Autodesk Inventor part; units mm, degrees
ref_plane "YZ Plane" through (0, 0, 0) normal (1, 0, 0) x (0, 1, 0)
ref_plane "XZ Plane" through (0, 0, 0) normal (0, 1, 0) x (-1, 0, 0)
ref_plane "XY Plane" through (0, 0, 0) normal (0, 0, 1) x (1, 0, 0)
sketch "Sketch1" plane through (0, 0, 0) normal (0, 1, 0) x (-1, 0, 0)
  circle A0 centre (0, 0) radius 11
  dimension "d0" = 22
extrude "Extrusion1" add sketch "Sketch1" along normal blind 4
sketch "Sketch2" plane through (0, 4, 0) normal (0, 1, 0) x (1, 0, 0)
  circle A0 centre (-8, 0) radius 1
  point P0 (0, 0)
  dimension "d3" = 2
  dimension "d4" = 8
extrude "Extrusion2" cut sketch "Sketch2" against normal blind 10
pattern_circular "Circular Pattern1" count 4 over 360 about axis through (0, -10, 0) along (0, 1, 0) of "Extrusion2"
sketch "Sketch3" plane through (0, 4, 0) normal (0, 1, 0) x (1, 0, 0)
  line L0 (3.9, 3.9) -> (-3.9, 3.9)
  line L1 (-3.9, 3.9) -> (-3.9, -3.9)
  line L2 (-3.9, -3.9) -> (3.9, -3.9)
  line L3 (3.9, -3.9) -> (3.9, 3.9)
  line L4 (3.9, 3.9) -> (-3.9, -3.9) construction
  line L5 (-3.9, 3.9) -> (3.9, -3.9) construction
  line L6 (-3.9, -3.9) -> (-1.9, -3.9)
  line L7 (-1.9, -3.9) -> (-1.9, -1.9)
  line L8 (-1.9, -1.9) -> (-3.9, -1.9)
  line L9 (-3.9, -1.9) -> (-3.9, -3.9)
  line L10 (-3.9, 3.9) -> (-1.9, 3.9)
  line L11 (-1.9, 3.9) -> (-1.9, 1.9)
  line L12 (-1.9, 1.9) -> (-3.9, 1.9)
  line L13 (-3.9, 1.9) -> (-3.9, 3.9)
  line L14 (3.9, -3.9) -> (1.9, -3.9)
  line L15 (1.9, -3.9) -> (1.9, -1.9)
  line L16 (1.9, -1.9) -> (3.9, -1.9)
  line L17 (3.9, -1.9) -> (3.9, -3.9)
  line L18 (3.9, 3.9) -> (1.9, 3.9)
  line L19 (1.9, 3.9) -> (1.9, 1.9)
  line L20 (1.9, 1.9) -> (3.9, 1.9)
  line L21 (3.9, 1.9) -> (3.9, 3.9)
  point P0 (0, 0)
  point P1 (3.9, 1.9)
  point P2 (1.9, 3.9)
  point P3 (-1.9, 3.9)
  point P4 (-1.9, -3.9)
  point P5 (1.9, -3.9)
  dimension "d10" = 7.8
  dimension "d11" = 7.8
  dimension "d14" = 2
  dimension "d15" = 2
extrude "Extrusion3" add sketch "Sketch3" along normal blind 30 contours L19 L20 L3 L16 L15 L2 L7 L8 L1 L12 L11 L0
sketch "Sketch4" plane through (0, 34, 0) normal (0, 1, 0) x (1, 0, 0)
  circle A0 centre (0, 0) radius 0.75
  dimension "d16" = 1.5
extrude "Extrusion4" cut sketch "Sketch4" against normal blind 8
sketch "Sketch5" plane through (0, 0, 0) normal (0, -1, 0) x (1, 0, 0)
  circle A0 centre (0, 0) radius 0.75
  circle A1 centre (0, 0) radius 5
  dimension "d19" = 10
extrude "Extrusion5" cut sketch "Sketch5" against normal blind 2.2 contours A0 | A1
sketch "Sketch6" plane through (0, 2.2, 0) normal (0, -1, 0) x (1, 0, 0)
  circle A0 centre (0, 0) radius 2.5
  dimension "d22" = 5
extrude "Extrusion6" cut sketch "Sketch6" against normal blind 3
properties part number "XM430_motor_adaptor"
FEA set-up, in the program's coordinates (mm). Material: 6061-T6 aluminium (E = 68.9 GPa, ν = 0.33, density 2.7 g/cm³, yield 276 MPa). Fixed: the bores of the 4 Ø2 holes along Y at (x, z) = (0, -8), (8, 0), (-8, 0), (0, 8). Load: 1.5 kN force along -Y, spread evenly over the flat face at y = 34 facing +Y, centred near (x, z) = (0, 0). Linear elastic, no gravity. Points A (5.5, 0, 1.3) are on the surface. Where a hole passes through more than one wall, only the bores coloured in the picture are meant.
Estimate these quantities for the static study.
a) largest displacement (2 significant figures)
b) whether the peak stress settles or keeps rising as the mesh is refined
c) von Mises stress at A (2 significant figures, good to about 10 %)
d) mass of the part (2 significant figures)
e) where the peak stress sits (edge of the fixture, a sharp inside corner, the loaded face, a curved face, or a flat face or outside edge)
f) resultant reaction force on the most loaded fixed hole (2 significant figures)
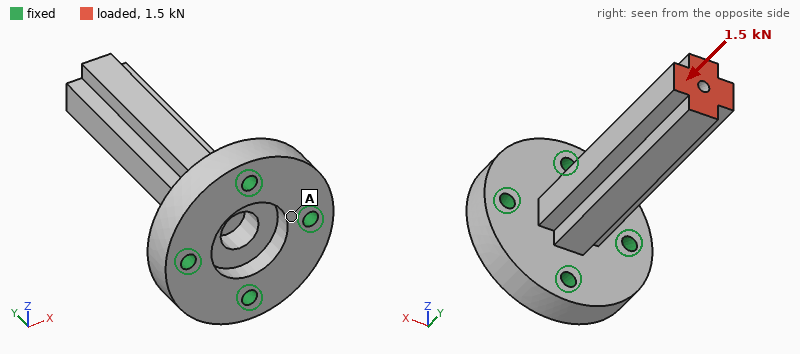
23 µm
keeps rising
18 MPa
6.9 g
edge of the fixture
420 N
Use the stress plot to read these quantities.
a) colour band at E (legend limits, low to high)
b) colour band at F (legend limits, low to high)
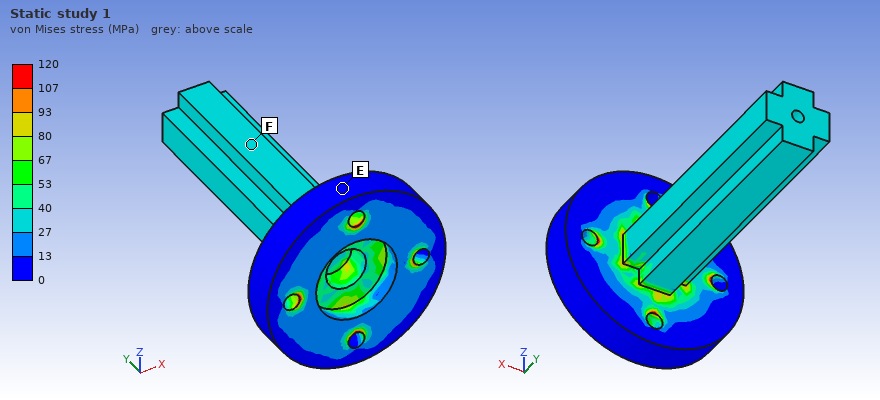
0 to 13 MPa
27 to 40 MPa
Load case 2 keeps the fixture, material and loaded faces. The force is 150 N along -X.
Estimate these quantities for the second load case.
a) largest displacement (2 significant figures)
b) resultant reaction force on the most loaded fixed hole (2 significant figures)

0.19 mm
390 N
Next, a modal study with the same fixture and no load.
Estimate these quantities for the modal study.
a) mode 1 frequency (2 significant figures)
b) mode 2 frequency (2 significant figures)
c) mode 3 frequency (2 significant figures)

4500 Hz
4500 Hz
21 kHz
